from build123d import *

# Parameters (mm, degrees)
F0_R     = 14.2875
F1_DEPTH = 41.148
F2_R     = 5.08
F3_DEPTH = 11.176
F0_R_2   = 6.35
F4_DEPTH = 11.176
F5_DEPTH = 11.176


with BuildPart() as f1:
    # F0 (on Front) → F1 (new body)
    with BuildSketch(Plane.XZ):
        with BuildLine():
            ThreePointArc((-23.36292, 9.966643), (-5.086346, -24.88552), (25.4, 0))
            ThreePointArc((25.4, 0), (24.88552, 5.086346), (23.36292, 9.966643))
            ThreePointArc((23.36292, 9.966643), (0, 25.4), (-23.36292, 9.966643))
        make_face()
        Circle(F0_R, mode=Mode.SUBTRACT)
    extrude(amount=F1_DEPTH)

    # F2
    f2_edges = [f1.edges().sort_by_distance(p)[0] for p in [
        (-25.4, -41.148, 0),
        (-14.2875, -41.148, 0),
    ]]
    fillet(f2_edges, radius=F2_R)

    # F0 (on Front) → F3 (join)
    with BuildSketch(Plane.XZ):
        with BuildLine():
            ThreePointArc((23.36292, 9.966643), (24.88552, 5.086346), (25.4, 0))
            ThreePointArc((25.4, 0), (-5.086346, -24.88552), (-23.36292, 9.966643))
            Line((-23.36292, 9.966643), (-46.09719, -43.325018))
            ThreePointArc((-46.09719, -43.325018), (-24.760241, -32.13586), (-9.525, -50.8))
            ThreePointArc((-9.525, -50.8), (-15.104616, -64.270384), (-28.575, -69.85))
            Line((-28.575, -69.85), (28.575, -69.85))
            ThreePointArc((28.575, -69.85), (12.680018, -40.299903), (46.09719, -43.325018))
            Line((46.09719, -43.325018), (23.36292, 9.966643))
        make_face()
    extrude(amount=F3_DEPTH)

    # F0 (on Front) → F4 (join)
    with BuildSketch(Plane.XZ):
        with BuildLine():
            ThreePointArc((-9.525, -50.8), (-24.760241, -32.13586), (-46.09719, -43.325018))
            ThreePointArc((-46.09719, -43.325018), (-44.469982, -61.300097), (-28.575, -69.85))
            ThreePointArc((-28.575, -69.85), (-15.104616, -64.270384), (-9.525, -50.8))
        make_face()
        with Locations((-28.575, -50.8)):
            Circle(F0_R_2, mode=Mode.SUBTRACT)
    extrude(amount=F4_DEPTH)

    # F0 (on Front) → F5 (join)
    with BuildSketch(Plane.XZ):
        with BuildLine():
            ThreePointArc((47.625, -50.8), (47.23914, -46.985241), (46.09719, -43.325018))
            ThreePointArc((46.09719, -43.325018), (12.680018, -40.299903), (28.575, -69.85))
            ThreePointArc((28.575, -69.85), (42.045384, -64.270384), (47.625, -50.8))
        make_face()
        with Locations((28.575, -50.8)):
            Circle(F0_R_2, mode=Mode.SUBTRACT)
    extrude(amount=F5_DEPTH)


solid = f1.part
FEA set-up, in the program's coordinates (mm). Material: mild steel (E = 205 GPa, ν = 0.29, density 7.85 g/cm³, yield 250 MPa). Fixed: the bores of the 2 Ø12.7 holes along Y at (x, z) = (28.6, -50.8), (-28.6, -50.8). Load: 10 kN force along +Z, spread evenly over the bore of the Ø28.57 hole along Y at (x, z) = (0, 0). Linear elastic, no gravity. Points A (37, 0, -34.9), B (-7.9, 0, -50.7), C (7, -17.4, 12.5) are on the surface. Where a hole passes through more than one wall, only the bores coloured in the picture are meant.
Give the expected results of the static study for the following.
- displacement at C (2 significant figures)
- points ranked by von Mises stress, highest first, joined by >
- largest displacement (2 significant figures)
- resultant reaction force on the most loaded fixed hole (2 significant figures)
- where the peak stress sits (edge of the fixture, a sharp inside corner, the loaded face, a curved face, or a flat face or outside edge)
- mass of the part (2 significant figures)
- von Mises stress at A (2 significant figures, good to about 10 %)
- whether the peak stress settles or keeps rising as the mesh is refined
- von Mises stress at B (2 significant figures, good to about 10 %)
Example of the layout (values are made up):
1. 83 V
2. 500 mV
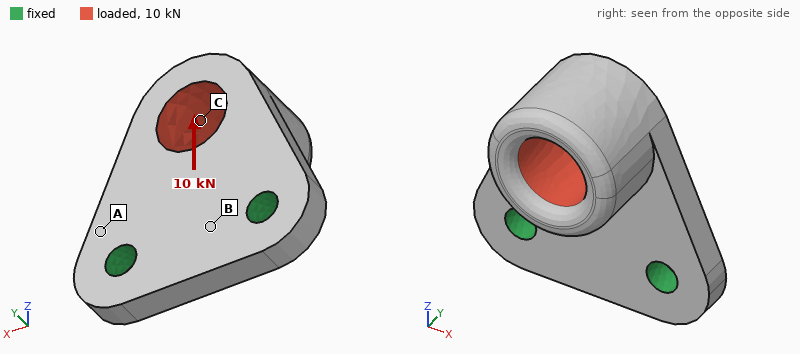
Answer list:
1. 0.10 mm
2. A > B > C
3. 0.15 mm
4. 5.2 kN
5. edge of the fixture
6. 810 g
7. 59 MPa
8. keeps rising
9. 20 MPa
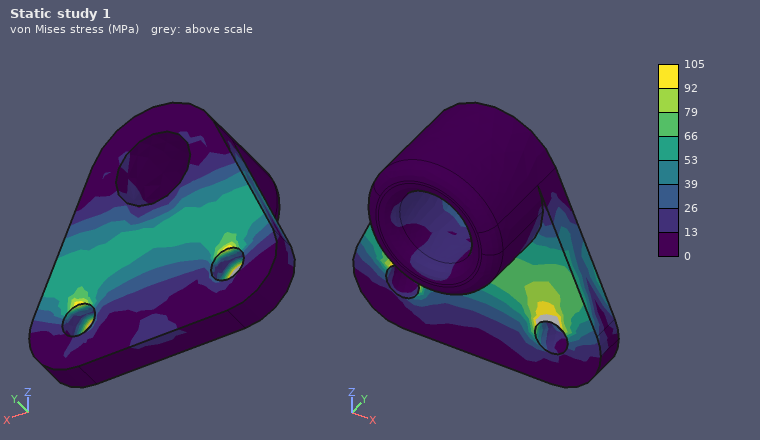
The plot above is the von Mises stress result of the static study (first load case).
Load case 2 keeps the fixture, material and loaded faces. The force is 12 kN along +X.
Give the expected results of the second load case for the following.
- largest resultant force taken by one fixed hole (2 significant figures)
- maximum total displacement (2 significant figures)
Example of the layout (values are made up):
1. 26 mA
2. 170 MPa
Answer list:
1. 11 kN
2. 46 µm
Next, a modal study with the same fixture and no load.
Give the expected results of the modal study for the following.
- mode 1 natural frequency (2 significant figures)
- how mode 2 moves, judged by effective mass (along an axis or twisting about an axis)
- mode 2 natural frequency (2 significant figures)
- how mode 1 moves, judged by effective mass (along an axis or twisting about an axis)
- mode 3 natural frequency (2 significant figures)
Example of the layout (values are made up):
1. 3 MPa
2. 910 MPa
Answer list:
1. 1400 Hz
2. along X
3. 3900 Hz
4. along Y
5. 6600 Hz
